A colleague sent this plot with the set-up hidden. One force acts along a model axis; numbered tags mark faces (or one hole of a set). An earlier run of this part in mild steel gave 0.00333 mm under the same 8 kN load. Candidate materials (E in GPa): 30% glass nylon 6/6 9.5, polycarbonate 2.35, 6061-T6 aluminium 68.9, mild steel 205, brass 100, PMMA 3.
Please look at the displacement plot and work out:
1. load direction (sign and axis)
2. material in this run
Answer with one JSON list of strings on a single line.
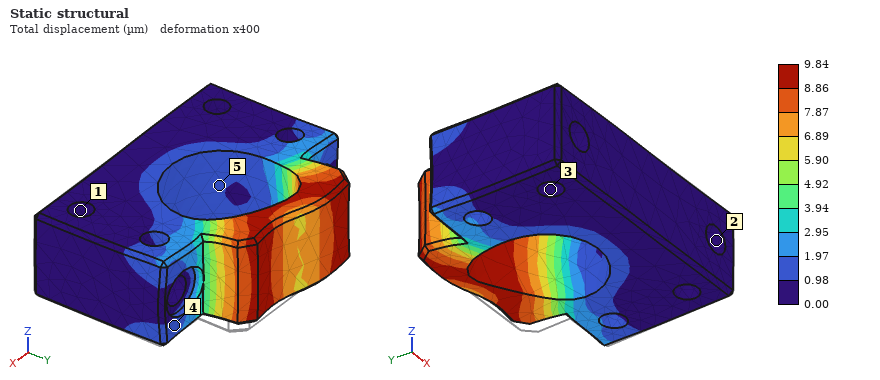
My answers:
["-X", "6061-T6 aluminium"]
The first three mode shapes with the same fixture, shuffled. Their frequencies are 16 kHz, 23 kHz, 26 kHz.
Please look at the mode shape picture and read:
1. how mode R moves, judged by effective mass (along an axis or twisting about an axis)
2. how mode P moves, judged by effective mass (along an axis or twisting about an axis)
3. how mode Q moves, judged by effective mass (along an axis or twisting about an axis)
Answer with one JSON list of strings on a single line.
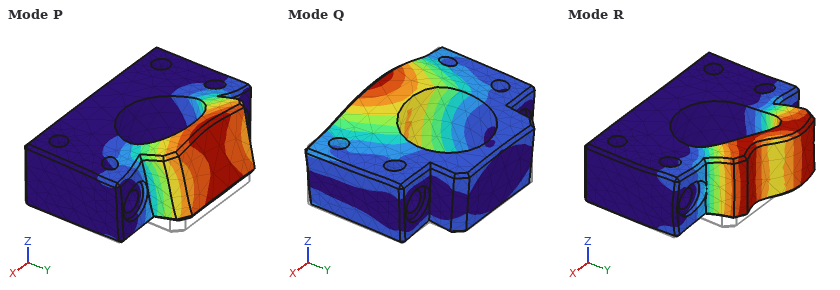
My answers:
["along X", "along Z", "along Z"]
